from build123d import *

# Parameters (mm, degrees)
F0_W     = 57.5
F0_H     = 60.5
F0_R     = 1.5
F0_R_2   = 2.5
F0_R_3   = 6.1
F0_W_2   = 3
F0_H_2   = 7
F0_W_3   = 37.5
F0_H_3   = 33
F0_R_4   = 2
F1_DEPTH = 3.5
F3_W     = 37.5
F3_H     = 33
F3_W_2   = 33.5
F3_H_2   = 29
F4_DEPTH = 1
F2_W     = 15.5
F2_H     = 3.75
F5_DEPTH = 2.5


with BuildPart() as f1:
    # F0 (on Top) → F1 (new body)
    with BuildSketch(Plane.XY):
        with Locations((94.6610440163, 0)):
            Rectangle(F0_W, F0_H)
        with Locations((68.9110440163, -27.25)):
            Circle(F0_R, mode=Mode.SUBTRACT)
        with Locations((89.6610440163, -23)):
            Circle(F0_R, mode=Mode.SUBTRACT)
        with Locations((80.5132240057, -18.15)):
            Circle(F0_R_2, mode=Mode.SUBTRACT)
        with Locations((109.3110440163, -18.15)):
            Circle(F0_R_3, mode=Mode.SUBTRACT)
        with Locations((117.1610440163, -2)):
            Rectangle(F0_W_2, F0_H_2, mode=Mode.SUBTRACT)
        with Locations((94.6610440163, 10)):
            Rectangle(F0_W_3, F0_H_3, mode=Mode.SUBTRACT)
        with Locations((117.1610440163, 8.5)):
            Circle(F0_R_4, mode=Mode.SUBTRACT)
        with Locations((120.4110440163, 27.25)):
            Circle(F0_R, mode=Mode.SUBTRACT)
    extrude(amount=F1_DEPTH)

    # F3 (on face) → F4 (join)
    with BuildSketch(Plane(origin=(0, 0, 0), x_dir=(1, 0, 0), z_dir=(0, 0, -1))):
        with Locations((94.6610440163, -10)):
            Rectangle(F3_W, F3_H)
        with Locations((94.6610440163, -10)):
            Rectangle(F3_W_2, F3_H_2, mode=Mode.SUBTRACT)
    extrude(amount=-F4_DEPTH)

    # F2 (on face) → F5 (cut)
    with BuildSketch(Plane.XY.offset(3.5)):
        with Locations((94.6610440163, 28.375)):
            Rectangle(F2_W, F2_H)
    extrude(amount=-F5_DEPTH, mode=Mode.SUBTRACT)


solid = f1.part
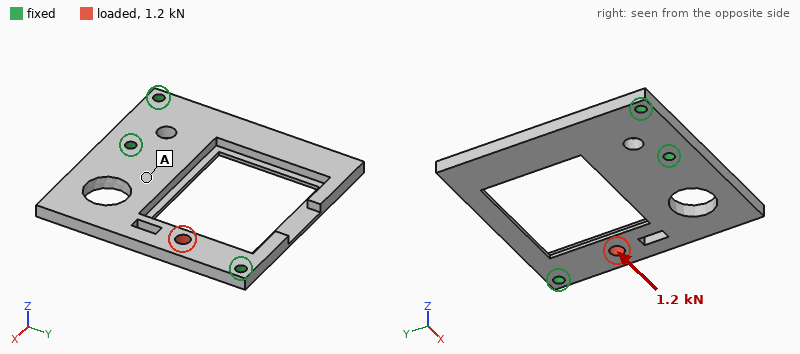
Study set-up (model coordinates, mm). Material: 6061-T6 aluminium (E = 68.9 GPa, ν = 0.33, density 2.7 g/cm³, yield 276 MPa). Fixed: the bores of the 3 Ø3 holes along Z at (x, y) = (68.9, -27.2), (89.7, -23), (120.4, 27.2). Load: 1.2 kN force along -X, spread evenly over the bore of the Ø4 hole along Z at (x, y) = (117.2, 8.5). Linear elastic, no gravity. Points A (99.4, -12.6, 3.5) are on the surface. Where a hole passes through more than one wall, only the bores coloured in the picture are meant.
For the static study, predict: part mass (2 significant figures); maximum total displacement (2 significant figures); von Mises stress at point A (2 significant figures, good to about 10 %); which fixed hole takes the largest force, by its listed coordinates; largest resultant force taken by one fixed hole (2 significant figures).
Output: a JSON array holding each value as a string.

["20 g", "52 µm", "16 MPa", "(120.4, 27.2)", "670 N"]
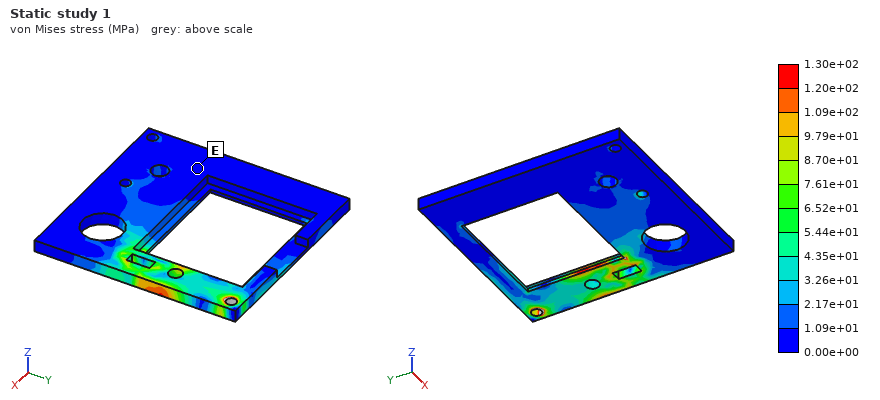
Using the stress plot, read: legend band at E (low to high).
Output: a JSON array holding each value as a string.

["0.00e+00 to 1.09e+01 MPa"]
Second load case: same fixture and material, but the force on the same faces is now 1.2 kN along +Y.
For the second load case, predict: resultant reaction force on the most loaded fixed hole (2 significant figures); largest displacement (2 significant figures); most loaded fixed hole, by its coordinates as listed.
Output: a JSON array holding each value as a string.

["1.1 kN", "15 µm", "(120.4, 27.2)"]
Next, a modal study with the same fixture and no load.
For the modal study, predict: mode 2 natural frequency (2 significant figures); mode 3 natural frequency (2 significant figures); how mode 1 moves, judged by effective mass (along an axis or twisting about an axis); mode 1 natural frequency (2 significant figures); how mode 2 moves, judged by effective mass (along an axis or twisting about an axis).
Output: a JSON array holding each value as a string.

["2800 Hz", "4700 Hz", "along Z", "1300 Hz", "along Z"]
